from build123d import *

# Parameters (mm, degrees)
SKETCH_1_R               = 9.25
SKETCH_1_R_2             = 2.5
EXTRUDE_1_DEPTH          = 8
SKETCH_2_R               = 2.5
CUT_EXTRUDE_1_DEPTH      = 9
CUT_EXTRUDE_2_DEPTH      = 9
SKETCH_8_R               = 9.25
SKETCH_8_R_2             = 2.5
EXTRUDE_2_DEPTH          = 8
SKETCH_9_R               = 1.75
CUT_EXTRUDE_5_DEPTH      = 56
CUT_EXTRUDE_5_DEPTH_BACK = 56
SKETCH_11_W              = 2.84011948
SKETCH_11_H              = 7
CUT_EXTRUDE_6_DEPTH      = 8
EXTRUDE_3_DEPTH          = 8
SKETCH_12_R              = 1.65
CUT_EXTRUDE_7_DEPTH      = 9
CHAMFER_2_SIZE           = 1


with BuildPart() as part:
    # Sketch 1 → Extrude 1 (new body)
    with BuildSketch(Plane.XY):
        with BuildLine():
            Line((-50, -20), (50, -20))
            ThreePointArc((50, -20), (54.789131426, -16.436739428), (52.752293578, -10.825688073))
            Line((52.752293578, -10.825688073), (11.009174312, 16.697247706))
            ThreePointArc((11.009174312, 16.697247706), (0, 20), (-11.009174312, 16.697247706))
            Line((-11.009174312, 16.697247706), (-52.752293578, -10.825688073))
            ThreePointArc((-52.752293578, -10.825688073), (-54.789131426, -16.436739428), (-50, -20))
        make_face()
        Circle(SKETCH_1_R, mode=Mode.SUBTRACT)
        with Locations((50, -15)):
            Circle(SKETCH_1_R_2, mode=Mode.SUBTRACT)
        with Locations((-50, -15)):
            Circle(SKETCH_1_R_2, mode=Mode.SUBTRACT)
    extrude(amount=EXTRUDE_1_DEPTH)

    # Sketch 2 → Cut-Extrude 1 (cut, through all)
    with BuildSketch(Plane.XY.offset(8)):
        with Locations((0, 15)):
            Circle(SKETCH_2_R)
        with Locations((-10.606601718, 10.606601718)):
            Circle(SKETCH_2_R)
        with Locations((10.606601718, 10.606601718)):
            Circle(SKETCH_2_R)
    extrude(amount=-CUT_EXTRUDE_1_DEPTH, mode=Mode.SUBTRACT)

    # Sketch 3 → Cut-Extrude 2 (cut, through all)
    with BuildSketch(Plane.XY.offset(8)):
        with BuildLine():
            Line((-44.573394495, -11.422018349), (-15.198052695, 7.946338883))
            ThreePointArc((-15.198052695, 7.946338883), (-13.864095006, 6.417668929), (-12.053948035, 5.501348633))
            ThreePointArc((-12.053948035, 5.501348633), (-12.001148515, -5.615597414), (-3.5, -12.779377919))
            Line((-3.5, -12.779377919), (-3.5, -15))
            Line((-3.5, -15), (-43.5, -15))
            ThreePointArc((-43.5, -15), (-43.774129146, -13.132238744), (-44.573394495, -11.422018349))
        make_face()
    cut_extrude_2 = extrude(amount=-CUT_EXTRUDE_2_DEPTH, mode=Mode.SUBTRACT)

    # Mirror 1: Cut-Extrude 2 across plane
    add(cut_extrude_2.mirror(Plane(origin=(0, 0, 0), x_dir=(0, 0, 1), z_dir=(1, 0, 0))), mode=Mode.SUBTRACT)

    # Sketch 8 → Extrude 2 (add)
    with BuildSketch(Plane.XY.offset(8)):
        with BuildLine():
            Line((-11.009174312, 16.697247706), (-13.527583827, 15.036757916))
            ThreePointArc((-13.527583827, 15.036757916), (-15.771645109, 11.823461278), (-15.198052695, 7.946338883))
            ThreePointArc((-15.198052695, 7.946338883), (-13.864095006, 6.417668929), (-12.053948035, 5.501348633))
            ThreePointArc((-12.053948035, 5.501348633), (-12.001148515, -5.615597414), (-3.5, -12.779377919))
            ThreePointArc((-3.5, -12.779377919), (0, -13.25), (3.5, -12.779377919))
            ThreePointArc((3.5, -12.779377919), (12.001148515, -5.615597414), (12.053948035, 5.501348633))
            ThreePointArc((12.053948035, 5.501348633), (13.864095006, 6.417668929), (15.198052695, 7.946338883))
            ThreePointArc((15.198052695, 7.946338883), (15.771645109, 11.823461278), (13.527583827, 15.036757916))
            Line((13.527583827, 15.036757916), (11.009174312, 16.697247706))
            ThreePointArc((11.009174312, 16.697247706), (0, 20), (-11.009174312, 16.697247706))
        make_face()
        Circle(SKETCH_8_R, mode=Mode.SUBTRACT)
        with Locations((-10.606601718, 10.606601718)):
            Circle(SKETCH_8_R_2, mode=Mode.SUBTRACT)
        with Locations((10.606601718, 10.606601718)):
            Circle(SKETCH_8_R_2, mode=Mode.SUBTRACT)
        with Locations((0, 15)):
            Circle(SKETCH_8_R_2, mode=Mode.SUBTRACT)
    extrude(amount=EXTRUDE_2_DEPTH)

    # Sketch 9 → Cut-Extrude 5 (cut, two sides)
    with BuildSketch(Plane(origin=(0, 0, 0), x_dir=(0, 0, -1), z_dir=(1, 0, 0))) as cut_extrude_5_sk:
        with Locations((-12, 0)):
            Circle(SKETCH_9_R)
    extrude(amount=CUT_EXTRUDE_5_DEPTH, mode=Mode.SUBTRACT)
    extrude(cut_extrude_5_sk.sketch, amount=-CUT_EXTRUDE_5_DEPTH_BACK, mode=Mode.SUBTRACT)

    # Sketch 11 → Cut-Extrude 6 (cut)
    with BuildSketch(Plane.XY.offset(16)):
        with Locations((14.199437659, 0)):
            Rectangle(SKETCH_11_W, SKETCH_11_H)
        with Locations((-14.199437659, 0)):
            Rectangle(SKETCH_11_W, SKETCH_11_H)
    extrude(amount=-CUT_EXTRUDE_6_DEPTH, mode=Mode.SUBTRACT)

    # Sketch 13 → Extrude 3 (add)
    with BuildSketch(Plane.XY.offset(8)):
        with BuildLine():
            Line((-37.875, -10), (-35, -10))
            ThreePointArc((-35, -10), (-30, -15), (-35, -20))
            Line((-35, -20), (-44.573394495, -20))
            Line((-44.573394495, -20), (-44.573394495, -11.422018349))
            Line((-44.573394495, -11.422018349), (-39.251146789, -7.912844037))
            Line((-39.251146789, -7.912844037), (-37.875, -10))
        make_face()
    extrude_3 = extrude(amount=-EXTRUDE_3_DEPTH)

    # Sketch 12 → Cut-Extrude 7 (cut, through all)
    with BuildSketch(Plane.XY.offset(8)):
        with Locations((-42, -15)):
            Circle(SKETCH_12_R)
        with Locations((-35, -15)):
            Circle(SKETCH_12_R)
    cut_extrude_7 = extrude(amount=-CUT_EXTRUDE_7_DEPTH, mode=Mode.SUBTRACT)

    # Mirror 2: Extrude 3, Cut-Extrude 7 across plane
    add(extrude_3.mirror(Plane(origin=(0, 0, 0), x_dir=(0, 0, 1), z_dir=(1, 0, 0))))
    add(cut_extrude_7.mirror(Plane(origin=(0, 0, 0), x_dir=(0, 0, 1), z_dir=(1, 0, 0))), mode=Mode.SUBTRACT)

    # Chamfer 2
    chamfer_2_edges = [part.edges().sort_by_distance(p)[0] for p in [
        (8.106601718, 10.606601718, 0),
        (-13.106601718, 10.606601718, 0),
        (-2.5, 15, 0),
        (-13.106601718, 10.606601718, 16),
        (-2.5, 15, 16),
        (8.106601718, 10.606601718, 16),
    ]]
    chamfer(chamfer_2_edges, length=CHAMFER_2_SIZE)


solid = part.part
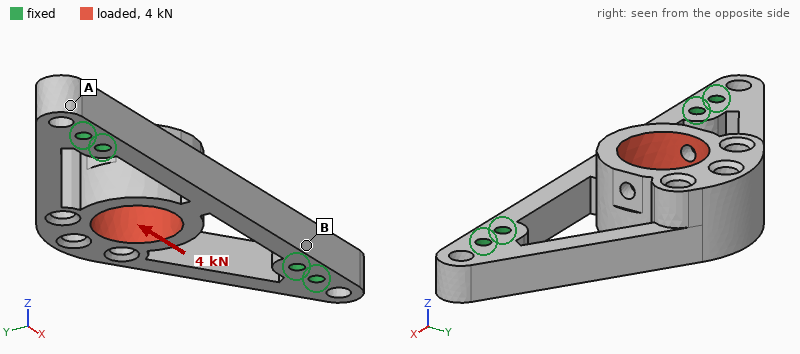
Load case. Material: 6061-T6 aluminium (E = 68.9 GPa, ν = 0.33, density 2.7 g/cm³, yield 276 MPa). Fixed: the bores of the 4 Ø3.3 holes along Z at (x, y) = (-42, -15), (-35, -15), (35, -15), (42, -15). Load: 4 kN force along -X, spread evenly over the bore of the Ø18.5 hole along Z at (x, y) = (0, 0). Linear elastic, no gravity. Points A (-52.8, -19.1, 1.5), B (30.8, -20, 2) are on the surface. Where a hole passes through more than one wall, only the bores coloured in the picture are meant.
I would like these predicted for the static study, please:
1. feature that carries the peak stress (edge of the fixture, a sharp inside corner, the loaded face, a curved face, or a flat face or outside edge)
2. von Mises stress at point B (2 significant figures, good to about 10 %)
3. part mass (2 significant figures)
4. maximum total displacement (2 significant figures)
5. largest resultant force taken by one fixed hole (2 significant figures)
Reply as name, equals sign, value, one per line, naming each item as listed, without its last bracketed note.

feature that carries the peak stress = a flat face or outside edge
von Mises stress at point B = 47 MPa
part mass = 43 g
maximum total displacement = 71 µm
largest resultant force taken by one fixed hole = 1.4 kN
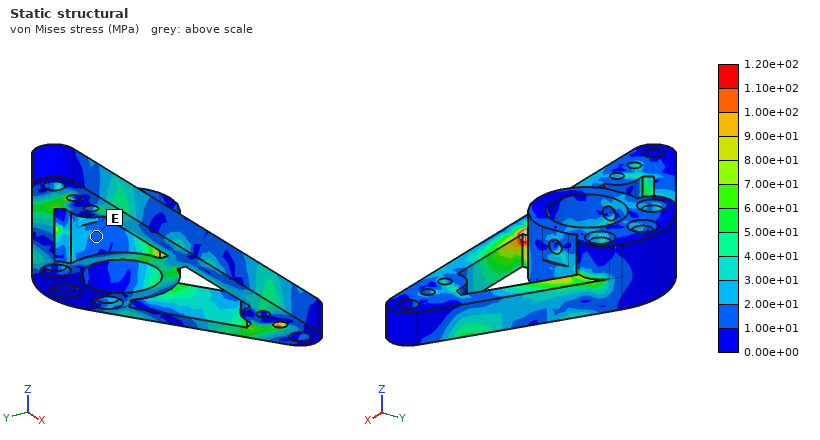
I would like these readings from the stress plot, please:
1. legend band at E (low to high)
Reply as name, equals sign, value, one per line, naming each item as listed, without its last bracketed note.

legend band at E = 1.00e+01 to 2.00e+01 MPa
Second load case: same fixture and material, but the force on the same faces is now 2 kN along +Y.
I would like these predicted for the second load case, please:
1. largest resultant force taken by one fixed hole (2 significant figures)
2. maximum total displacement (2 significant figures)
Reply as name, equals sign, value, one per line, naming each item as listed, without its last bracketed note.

largest resultant force taken by one fixed hole = 1.5 kN
maximum total displacement = 0.20 mm
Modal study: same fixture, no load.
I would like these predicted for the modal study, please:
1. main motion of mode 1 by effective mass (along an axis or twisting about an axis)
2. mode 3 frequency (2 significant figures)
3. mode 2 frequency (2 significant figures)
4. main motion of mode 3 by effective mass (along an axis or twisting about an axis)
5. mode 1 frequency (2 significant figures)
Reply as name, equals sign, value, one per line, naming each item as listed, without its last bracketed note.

main motion of mode 1 by effective mass = along Z
mode 3 frequency = 6700 Hz
mode 2 frequency = 5400 Hz
main motion of mode 3 by effective mass = along Y
mode 1 frequency = 2100 Hz
